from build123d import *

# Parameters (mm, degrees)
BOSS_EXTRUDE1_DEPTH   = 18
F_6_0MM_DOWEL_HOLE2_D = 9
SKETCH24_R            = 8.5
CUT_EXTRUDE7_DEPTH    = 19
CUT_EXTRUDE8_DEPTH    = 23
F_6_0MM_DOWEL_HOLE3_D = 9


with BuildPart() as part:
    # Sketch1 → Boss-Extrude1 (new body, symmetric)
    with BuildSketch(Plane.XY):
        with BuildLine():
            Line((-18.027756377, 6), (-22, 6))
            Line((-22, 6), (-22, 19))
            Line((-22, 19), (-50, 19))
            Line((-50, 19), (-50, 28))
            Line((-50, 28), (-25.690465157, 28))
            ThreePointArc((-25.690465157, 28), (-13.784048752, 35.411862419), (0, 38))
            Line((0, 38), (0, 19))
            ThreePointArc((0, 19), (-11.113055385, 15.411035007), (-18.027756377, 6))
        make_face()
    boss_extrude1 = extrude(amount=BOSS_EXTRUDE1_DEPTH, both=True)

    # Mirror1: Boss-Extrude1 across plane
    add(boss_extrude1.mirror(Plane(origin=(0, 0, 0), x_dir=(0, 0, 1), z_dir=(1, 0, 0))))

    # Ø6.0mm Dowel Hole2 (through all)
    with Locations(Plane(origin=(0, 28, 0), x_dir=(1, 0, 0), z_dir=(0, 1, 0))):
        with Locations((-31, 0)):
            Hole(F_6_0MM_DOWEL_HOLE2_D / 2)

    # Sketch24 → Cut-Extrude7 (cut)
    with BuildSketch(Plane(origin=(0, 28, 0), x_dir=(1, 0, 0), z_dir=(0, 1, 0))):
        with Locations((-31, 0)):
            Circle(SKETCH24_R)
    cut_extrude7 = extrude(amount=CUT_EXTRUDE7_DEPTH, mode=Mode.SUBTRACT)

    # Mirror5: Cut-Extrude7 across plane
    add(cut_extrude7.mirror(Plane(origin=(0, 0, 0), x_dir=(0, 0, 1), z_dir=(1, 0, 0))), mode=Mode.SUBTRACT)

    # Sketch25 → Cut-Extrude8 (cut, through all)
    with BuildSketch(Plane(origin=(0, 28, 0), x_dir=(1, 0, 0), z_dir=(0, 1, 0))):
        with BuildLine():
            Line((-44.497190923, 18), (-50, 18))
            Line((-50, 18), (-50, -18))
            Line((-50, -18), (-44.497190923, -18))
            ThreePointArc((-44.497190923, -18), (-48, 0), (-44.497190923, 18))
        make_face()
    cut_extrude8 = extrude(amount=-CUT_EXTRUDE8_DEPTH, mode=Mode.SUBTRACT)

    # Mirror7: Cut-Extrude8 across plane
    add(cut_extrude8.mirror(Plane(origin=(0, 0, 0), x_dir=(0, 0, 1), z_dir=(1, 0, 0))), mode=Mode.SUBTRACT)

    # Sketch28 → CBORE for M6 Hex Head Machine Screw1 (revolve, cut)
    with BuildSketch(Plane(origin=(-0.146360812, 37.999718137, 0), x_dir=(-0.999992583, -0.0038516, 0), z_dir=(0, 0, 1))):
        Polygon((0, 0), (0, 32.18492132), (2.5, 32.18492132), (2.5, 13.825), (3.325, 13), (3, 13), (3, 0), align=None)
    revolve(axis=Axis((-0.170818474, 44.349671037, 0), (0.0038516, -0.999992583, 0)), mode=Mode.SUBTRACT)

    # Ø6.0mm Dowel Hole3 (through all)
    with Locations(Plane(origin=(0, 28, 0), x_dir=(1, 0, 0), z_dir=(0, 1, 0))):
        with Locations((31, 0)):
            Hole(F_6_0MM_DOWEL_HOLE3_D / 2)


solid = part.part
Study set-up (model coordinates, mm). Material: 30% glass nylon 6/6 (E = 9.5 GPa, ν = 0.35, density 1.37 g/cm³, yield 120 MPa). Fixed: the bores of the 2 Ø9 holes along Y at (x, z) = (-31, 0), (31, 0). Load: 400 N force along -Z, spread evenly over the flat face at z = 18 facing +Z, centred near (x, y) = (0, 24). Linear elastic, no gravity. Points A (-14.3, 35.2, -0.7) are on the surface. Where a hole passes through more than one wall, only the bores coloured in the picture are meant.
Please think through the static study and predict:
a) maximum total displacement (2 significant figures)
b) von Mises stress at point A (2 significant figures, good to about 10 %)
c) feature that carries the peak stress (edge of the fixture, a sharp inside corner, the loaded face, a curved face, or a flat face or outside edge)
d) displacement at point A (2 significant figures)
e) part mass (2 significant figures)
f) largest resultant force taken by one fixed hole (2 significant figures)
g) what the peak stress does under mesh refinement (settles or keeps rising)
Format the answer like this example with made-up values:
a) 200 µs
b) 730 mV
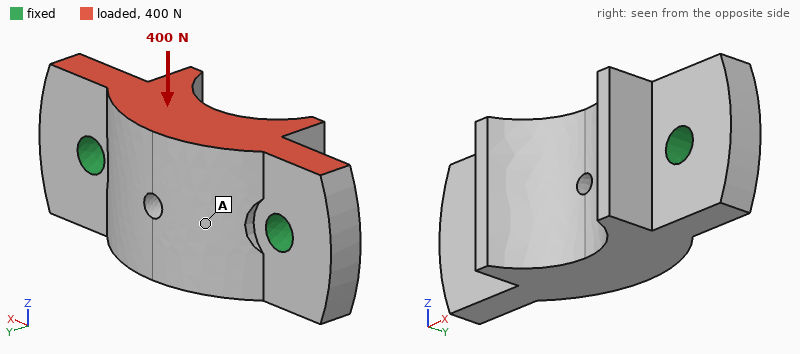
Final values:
a) 4.4 µm
b) 0.43 MPa
c) edge of the fixture
d) 3.0 µm
e) 68 g
f) 200 N
g) keeps rising
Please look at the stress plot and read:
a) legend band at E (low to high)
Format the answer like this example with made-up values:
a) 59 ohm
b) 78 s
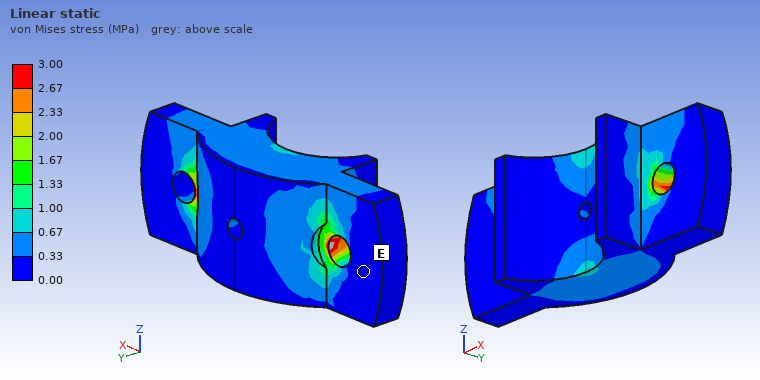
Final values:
a) 0.00 to 0.33 MPa
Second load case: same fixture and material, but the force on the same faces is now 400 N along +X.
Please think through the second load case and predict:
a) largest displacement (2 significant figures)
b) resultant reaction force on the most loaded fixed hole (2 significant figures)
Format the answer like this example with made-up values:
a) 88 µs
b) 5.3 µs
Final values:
a) 4.8 µm
b) 230 N
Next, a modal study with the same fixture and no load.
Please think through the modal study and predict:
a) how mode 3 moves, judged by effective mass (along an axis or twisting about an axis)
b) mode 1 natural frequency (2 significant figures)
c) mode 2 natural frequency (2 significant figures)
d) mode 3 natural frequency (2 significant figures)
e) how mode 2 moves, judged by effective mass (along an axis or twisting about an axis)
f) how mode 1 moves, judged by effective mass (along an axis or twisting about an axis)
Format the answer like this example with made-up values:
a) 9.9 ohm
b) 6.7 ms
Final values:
a) along Z
b) 4700 Hz
c) 6000 Hz
d) 7600 Hz
e) along Y
f) twisting about X
